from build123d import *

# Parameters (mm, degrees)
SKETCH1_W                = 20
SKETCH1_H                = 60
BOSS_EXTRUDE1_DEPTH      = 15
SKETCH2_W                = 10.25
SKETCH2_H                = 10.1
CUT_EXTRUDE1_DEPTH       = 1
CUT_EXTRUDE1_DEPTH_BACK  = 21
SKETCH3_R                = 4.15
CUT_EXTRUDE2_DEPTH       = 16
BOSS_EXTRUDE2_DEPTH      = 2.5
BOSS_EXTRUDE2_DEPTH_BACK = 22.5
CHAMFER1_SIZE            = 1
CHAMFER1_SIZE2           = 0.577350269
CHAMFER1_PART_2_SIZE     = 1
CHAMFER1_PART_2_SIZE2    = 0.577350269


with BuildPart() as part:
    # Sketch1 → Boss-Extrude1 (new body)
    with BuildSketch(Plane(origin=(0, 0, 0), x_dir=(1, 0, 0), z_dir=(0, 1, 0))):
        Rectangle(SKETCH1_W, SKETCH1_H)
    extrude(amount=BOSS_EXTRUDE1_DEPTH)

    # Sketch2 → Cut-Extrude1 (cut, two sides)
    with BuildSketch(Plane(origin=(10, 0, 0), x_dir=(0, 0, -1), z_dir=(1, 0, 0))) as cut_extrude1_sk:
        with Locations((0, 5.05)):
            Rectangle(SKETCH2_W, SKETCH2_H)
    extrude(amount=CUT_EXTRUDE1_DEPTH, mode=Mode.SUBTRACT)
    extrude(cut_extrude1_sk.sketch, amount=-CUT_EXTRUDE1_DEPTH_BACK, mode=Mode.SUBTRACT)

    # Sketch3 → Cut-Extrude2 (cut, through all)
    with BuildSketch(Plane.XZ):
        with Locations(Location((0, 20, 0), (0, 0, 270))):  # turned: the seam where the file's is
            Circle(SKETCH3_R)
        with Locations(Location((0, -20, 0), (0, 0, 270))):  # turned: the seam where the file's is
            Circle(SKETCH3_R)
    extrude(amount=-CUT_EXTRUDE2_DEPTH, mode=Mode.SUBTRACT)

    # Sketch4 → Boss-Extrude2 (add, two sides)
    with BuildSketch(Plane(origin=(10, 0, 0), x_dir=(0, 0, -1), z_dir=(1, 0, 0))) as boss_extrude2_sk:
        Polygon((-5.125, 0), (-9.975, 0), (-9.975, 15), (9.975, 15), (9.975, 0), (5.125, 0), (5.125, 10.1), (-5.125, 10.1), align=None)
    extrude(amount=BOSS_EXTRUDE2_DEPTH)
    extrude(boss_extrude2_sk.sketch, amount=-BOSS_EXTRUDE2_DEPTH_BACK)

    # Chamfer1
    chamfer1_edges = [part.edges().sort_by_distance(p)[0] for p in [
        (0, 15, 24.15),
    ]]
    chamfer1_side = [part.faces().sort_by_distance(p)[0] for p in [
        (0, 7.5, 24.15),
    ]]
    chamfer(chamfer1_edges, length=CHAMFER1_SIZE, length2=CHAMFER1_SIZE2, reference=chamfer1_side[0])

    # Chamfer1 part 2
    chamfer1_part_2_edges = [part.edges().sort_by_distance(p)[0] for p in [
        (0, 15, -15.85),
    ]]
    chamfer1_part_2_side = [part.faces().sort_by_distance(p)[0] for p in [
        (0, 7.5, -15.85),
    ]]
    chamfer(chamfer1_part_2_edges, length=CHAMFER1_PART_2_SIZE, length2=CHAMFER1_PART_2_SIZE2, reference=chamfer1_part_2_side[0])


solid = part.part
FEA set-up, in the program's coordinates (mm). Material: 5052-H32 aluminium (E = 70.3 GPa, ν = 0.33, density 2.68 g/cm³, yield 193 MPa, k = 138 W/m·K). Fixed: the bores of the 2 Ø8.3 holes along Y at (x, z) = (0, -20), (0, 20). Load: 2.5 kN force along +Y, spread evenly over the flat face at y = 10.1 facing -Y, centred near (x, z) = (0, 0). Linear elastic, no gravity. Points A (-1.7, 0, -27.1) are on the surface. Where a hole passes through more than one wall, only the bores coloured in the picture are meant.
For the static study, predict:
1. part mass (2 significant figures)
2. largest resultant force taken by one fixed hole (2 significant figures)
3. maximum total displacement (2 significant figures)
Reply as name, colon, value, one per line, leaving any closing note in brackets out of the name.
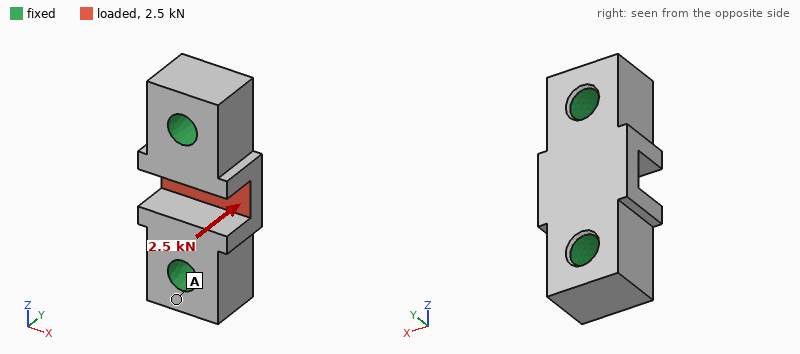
part mass: 41 g
largest resultant force taken by one fixed hole: 1.5 kN
maximum total displacement: 8.4 µm
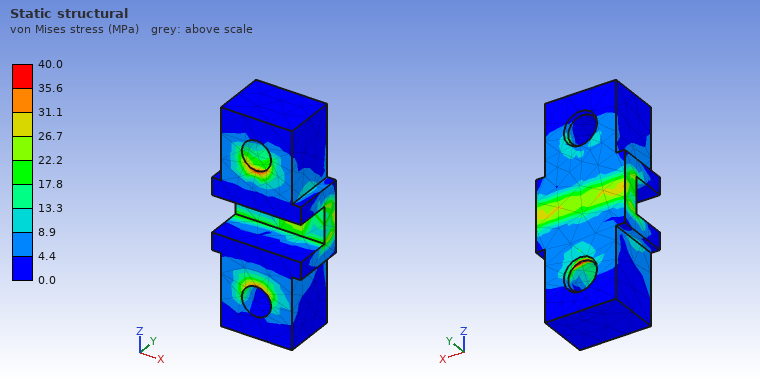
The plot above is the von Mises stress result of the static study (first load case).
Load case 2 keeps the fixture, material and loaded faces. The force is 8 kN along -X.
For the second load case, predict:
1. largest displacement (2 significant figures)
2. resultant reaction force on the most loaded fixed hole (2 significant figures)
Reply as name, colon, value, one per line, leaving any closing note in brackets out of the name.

largest displacement: 24 µm
resultant reaction force on the most loaded fixed hole: 4.0 kN
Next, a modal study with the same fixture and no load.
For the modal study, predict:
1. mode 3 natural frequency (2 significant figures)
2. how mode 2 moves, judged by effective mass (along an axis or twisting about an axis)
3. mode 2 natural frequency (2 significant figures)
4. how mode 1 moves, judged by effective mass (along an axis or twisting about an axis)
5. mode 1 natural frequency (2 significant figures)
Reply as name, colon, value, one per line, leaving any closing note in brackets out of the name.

mode 3 natural frequency: 39 kHz
how mode 2 moves, judged by effective mass: along Y
mode 2 natural frequency: 35 kHz
how mode 1 moves, judged by effective mass: along X
mode 1 natural frequency: 32 kHz
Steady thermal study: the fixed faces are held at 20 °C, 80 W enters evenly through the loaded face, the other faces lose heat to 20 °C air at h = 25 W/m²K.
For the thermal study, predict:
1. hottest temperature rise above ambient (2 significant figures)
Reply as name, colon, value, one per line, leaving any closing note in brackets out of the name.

hottest temperature rise above ambient: 27 K
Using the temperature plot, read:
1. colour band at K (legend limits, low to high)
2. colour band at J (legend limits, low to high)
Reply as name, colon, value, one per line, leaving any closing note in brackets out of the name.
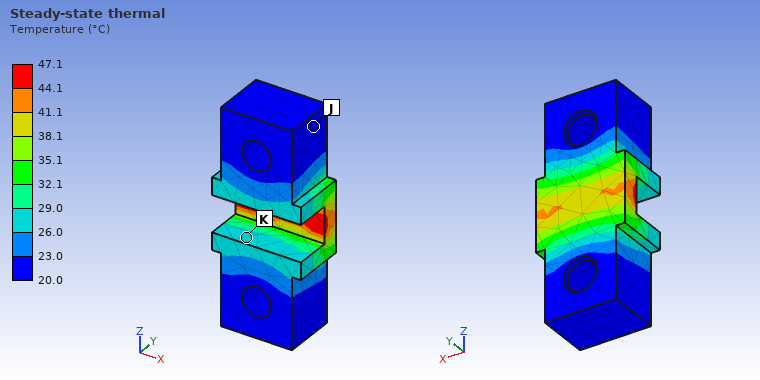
colour band at K: 26.0 to 29.0 °C
colour band at J: 20.0 to 23.0 °C
